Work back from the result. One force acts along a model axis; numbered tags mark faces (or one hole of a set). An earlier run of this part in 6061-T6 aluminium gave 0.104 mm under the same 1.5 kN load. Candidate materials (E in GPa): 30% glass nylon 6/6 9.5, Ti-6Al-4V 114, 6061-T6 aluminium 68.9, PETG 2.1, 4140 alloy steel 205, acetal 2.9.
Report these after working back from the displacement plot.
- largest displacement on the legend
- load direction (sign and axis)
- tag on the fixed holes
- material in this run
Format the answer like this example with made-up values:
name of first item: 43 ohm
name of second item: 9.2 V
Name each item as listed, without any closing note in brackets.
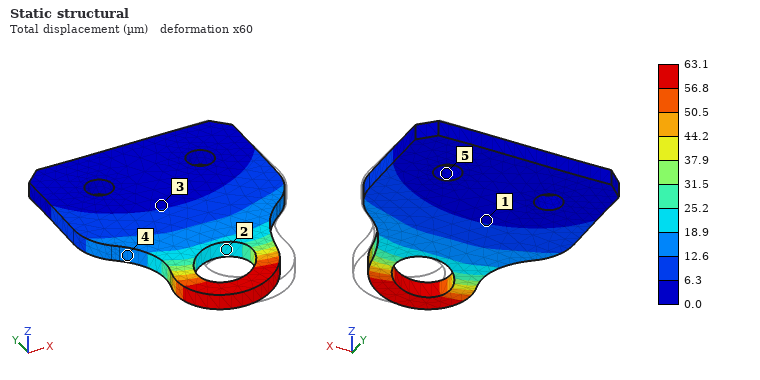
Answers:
largest displacement on the legend: 63.1 µm
load direction: -X
tag on the fixed holes: 5
material in this run: Ti-6Al-4V
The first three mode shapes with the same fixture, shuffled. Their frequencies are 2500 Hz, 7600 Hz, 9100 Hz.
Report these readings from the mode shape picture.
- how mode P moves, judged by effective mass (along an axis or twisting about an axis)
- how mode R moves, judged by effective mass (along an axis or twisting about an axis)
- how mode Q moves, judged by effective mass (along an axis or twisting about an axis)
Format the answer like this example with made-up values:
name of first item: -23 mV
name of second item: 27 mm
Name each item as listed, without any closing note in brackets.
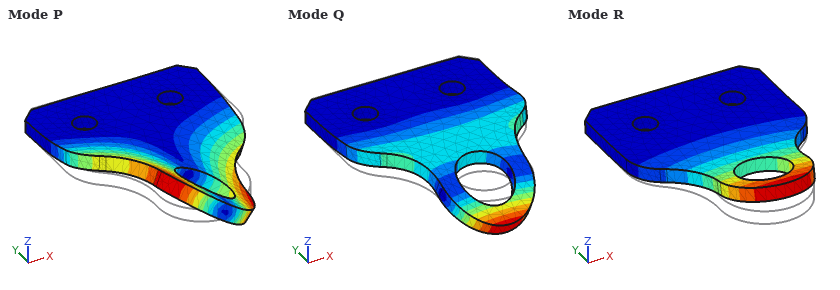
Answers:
how mode P moves, judged by effective mass: twisting about Y
how mode R moves, judged by effective mass: along Z
how mode Q moves, judged by effective mass: along Z
